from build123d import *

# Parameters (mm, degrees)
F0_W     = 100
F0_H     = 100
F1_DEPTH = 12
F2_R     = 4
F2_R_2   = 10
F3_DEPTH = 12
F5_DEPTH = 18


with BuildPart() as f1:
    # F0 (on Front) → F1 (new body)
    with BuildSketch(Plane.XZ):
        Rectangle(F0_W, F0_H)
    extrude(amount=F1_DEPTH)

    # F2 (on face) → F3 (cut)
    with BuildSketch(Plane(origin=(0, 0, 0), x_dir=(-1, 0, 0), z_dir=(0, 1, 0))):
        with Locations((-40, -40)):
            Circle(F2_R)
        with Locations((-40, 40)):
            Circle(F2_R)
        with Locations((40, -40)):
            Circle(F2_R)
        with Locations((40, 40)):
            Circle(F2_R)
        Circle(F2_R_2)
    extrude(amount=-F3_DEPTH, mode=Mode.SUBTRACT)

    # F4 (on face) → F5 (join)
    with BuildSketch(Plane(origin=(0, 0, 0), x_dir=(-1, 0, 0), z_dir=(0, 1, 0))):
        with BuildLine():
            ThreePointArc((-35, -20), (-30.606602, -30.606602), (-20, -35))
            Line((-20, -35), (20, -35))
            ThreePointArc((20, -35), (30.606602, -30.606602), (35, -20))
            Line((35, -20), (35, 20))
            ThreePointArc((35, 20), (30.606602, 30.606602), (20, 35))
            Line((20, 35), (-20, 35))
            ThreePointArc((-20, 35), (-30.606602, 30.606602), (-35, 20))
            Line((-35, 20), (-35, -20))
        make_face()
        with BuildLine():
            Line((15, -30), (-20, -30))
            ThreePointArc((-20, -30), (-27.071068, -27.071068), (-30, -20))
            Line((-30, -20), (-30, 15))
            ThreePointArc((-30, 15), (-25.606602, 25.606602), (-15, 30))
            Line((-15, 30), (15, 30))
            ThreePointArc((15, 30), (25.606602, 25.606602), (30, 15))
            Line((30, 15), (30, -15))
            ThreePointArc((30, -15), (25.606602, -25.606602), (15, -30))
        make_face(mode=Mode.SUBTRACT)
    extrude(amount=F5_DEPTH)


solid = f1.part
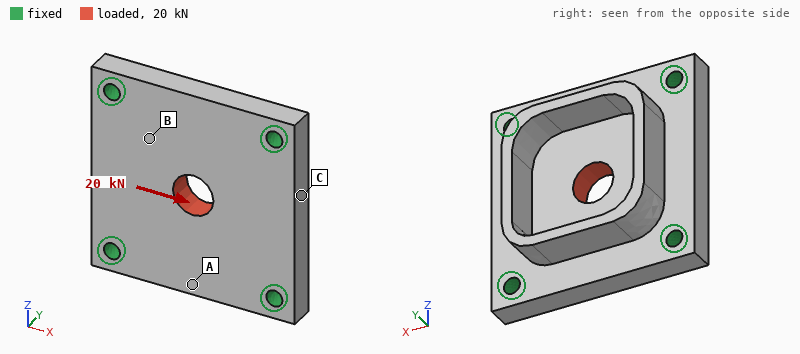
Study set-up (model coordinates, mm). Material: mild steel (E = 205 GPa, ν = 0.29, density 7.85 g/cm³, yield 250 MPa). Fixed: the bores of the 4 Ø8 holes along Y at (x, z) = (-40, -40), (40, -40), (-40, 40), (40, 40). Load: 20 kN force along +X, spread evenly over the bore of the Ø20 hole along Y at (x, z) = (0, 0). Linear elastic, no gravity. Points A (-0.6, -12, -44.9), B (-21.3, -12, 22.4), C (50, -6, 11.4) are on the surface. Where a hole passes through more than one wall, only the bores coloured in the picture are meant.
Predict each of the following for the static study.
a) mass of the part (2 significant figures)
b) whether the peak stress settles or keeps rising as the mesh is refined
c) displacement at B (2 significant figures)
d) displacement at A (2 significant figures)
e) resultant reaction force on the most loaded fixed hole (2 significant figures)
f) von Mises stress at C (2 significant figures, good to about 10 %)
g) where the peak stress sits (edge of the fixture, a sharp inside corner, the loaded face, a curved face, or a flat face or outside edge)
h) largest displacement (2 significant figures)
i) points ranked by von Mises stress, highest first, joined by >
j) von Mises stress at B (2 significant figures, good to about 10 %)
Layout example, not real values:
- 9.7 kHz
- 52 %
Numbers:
- 1.1 kg
- keeps rising
- 2.8 µm
- 1.3 µm
- 5.6 kN
- 11 MPa
- edge of the fixture
- 6.0 µm
- B > C > A
- 19 MPa
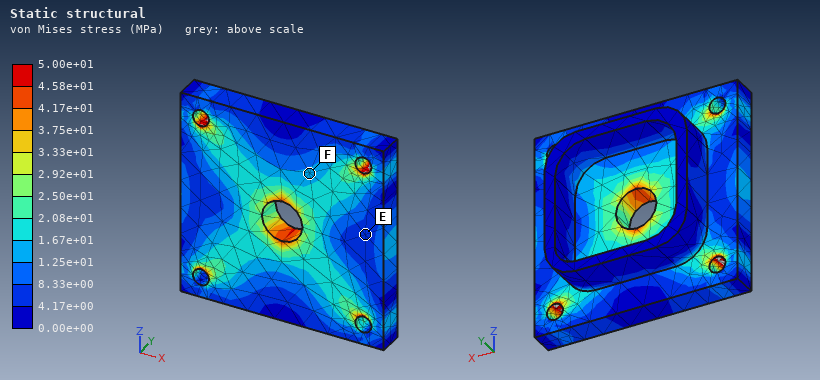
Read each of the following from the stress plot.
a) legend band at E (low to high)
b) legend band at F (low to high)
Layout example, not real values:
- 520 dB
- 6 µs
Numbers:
- 4.17e+00 to 8.33e+00 MPa
- 1.25e+01 to 1.67e+01 MPa
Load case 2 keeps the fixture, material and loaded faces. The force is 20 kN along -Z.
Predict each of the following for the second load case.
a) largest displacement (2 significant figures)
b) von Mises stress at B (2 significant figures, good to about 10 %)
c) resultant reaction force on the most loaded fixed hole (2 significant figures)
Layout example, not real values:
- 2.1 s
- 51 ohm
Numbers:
- 6.0 µm
- 19 MPa
- 5.6 kN
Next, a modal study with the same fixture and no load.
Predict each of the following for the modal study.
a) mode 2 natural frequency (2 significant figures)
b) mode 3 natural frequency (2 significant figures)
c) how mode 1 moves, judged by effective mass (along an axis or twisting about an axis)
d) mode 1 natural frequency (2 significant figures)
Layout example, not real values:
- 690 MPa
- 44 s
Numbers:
- 9900 Hz
- 9900 Hz
- along Y
- 6900 Hz
